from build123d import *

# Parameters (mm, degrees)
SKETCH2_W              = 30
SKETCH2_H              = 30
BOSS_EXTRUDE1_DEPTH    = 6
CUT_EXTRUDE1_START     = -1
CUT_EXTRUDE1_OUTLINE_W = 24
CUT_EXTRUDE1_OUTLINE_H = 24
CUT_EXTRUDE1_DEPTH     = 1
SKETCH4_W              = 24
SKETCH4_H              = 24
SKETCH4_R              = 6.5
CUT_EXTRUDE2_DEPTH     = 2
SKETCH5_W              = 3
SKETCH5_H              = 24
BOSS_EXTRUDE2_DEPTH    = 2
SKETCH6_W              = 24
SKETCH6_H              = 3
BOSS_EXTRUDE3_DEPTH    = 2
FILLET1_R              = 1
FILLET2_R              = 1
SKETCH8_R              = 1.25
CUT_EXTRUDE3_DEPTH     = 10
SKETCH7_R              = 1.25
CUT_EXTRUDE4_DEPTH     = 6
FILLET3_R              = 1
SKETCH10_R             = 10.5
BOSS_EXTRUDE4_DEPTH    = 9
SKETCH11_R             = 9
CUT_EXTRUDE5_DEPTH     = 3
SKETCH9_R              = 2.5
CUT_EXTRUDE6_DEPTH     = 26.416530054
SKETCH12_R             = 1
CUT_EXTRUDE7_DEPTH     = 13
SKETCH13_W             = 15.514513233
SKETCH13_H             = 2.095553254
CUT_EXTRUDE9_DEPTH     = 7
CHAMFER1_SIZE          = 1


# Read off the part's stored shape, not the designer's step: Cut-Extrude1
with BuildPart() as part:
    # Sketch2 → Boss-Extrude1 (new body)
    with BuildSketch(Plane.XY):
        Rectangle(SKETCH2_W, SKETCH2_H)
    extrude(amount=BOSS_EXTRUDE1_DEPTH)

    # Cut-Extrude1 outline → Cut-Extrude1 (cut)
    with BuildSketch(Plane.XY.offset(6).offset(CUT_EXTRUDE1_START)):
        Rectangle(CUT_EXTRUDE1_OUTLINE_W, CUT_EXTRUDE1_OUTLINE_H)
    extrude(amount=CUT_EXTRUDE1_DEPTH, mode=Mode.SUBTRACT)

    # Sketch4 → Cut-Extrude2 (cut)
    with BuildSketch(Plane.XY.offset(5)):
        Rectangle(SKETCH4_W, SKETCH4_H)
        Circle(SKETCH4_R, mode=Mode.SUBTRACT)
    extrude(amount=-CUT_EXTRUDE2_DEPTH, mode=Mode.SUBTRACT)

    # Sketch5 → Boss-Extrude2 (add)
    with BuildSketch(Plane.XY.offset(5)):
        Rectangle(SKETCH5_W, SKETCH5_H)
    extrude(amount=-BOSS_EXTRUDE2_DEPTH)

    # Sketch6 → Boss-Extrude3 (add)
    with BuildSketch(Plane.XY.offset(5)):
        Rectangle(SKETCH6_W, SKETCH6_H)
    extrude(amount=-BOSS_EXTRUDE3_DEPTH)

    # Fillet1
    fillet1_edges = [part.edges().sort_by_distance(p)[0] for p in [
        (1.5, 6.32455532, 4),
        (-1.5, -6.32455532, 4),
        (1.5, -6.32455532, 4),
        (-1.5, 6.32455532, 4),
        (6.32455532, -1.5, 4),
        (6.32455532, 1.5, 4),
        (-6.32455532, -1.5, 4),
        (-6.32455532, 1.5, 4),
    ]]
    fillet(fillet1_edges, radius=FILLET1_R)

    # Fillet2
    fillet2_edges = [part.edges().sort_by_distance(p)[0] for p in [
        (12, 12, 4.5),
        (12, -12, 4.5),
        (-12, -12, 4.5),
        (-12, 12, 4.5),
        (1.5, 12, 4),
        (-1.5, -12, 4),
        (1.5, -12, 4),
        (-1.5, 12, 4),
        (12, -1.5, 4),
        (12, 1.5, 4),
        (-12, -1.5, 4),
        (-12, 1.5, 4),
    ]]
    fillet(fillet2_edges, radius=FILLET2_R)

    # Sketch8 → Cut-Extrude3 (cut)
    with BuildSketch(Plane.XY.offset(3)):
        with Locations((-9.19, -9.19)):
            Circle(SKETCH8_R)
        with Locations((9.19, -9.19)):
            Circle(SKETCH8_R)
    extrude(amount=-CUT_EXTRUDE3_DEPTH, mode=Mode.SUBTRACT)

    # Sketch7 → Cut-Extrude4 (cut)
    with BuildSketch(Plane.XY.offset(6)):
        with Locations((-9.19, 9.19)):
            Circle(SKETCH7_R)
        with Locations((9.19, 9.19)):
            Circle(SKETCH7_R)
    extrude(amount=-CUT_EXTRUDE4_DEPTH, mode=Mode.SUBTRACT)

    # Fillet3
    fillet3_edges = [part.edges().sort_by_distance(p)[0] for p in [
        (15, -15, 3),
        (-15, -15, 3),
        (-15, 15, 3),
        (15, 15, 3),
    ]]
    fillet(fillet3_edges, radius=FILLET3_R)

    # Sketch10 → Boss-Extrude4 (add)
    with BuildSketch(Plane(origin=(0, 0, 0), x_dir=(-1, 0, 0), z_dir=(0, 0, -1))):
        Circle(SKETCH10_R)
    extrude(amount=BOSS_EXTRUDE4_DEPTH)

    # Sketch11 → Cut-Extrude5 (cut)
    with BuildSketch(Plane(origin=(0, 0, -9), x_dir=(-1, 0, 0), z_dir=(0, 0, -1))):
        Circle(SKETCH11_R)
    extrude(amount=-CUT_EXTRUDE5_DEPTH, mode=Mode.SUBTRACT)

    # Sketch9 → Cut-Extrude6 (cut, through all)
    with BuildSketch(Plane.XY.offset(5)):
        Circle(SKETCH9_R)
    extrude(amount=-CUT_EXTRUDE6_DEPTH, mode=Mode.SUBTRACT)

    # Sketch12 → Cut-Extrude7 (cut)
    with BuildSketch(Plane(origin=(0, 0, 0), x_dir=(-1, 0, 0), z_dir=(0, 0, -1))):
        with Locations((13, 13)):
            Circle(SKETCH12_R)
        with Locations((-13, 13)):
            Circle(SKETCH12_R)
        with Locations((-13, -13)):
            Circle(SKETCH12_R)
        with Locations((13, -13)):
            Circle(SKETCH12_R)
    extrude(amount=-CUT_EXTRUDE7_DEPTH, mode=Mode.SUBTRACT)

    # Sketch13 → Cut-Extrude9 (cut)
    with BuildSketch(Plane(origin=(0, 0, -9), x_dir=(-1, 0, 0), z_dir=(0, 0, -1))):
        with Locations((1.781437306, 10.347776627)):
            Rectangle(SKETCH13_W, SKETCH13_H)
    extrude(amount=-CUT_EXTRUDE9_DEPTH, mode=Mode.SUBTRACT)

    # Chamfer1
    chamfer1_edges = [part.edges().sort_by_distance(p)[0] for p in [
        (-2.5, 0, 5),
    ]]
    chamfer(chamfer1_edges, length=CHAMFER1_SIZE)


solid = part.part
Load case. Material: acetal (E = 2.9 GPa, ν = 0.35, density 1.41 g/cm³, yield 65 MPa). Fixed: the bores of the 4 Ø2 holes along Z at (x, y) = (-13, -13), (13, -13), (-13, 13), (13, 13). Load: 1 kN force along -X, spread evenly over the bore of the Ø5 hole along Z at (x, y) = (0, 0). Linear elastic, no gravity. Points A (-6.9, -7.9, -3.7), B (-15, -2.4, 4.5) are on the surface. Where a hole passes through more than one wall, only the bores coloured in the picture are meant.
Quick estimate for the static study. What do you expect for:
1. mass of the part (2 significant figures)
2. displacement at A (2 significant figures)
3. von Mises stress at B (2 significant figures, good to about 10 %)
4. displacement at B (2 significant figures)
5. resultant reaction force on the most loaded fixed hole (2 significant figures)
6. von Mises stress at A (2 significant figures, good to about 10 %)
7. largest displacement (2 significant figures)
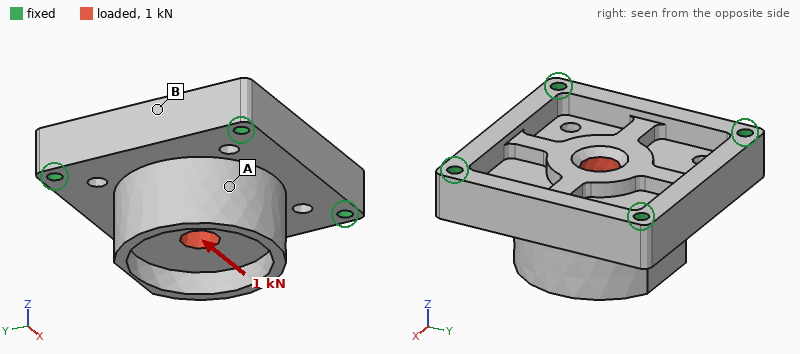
8.5 g
72 µm
6.5 MPa
59 µm
280 N
2.7 MPa
92 µm
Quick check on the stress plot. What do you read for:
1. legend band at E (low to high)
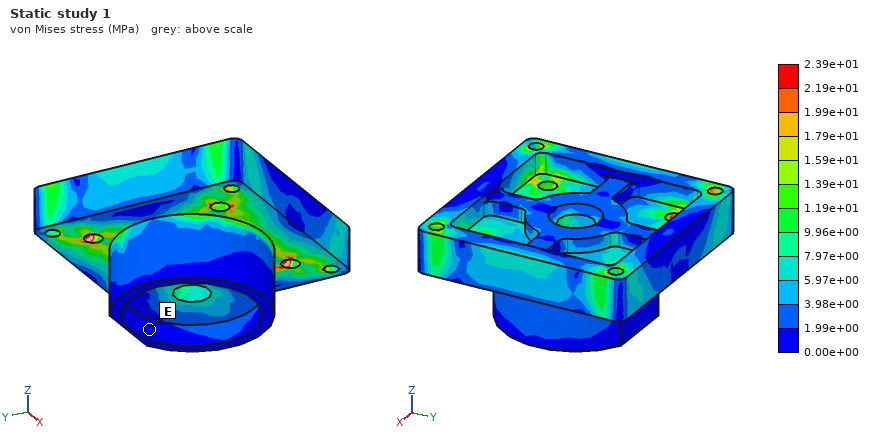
0.00e+00 to 1.99e+00 MPa
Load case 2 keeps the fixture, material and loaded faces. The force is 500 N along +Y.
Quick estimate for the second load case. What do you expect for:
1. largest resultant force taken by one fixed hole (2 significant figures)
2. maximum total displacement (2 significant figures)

140 N
46 µm
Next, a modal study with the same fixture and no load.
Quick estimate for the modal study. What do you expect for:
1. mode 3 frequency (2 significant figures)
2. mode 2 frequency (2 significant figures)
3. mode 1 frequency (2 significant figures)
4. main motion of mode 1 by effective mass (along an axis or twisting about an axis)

7000 Hz
6900 Hz
5100 Hz
along Z
